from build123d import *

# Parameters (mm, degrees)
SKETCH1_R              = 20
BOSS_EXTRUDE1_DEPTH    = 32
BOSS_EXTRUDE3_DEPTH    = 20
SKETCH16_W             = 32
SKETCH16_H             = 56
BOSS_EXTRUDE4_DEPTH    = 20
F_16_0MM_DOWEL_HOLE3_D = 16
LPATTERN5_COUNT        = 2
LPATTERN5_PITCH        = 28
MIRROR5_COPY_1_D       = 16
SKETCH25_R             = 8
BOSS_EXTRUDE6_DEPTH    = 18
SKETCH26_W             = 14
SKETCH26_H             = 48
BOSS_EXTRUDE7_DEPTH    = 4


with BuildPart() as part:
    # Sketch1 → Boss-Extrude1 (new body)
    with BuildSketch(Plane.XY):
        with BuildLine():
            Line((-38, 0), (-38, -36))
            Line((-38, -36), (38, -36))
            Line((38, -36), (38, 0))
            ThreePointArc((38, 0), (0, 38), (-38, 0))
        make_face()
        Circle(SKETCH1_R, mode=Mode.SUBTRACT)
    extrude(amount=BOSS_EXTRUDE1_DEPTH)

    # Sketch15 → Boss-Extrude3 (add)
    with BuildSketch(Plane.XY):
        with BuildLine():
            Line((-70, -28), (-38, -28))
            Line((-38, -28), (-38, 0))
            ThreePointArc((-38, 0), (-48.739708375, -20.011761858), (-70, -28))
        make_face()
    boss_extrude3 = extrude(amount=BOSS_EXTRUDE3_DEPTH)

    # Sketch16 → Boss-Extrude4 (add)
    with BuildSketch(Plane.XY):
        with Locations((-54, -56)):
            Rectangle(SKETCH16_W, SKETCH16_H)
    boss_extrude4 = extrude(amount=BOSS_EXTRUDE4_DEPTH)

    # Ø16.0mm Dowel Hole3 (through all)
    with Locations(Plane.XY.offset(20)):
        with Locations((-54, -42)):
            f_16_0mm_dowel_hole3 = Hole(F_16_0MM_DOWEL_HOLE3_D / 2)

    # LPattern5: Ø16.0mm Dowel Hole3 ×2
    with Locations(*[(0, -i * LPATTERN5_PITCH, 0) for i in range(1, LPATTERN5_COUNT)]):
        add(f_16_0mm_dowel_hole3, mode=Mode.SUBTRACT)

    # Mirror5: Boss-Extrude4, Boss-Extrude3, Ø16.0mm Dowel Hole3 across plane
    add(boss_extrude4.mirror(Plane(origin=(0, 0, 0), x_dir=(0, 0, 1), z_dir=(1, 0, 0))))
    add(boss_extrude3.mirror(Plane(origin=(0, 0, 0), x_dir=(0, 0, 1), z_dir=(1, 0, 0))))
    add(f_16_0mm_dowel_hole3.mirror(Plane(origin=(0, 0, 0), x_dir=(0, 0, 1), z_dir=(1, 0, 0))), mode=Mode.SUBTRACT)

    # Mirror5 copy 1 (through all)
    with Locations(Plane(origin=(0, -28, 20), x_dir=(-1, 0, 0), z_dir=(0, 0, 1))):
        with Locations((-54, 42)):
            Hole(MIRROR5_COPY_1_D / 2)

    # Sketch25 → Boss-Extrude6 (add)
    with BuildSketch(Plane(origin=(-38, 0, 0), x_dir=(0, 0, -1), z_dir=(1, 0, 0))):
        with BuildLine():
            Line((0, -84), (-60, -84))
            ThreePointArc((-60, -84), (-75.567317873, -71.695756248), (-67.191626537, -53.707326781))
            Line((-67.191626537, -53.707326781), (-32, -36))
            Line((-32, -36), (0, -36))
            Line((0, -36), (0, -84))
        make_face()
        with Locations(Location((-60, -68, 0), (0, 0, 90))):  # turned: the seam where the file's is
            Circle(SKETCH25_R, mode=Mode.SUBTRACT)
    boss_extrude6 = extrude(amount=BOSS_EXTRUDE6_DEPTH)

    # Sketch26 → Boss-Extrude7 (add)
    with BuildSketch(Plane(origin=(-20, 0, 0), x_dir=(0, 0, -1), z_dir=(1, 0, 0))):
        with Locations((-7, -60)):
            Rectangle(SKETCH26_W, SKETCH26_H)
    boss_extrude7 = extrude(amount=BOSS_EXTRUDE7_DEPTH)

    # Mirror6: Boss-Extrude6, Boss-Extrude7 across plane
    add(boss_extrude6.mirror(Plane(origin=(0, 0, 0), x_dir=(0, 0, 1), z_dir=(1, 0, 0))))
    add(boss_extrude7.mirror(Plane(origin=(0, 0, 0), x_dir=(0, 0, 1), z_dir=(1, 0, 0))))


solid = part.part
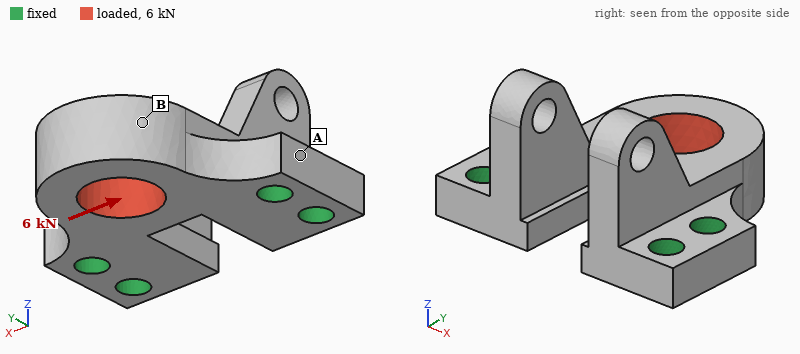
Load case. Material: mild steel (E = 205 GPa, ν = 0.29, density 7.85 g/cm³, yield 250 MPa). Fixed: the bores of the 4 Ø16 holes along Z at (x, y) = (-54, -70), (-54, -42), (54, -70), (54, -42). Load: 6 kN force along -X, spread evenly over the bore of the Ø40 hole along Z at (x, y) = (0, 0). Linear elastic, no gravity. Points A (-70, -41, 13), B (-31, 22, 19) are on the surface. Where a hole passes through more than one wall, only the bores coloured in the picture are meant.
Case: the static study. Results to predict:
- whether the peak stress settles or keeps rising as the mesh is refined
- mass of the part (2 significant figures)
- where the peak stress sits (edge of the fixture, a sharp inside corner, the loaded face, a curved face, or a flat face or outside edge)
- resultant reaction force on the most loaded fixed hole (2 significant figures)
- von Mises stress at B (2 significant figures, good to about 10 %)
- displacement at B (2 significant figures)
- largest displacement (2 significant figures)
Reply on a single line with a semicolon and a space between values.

keeps rising; 2.3 kg; edge of the fixture; 3.7 kN; 4.6 MPa; 4.5 µm; 4.9 µm
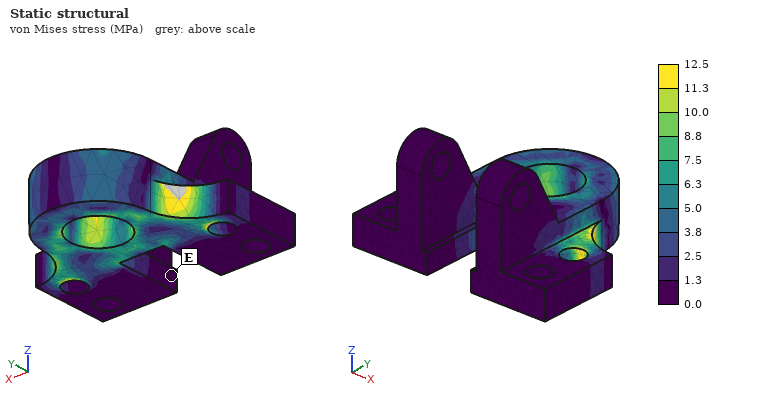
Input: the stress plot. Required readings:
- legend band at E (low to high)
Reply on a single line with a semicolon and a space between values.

0.0 to 1.3 MPa
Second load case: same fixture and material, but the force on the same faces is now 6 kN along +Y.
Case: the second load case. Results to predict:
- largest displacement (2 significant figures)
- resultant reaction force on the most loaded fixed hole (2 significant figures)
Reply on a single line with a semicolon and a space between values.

3.3 µm; 2.0 kN
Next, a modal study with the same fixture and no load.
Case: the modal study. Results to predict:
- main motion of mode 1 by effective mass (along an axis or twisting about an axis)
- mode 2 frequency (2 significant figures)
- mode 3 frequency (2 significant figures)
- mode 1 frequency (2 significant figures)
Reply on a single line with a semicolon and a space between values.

along Z; 4200 Hz; 4300 Hz; 3000 Hz
